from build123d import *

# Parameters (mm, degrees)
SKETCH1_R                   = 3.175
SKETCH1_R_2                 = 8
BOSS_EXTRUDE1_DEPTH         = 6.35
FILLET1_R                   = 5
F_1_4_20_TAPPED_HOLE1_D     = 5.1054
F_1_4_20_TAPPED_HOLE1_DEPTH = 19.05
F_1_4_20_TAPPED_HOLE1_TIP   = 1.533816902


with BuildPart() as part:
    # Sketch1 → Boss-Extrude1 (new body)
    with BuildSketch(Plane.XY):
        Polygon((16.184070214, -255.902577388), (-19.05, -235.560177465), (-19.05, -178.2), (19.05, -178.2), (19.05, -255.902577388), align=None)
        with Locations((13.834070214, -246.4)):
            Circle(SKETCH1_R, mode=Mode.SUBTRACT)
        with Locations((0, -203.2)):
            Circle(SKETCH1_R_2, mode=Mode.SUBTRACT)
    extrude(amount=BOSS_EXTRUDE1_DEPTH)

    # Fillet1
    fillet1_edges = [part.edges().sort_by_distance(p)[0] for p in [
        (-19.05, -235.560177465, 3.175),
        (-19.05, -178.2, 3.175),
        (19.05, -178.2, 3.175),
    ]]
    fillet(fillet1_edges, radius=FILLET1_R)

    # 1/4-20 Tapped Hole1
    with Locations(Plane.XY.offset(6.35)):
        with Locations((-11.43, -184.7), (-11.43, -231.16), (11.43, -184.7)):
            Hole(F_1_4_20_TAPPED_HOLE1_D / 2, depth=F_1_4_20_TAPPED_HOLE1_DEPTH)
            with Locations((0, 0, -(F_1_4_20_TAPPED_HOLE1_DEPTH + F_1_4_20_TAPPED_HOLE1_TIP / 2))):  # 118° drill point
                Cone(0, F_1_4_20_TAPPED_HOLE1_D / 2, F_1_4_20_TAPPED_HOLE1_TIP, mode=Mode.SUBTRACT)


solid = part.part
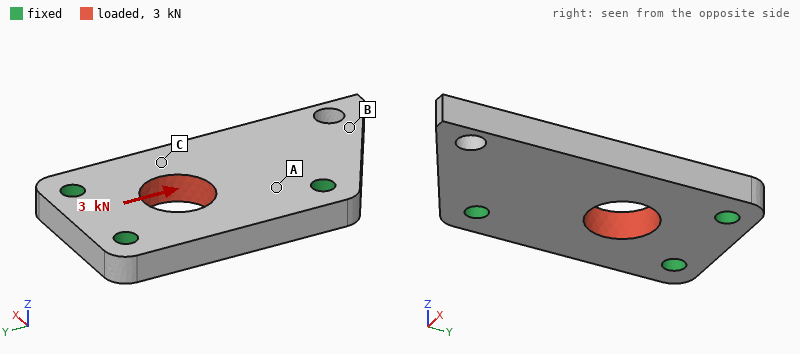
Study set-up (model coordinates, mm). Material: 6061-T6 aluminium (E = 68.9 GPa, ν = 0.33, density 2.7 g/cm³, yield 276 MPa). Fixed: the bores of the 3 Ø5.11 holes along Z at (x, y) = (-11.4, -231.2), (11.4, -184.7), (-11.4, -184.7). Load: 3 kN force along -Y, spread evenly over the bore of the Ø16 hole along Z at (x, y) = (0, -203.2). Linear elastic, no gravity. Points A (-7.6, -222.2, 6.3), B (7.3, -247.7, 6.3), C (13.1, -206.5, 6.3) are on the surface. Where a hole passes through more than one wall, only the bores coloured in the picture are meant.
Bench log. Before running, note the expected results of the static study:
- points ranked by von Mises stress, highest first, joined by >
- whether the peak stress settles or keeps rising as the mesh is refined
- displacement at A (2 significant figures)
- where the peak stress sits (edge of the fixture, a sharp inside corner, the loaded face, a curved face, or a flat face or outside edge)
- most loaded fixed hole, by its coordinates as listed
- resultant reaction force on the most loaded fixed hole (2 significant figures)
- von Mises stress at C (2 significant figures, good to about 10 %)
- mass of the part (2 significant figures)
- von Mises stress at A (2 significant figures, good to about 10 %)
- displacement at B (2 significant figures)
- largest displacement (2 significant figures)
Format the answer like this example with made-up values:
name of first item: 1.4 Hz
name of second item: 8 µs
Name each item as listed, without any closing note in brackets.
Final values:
points ranked by von Mises stress, highest first, joined by >: A > C > B
whether the peak stress settles or keeps rising as the mesh is refined: keeps rising
displacement at A: 1.5 µm
where the peak stress sits: edge of the fixture
most loaded fixed hole, by its coordinates as listed: (11.4, -184.7)
resultant reaction force on the most loaded fixed hole: 1.2 kN
von Mises stress at C: 5.2 MPa
mass of the part: 39 g
von Mises stress at A: 9.6 MPa
displacement at B: 3.5 µm
largest displacement: 5.1 µm
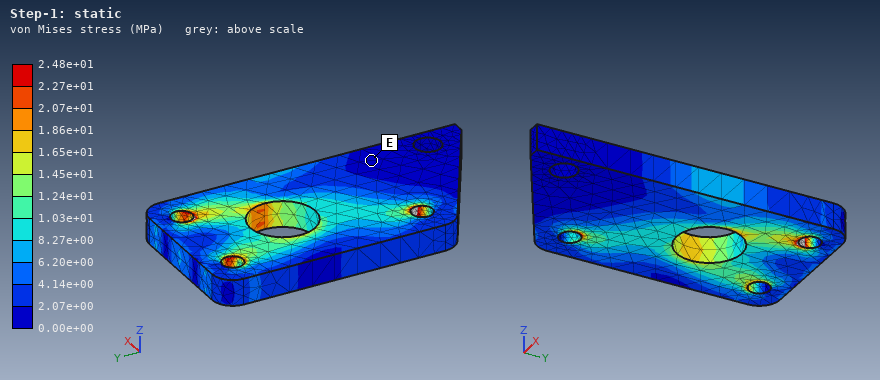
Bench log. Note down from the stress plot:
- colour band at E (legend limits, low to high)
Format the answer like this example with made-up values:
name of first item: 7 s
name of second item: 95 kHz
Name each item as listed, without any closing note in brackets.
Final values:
colour band at E: 0.00e+00 to 2.07e+00 MPa
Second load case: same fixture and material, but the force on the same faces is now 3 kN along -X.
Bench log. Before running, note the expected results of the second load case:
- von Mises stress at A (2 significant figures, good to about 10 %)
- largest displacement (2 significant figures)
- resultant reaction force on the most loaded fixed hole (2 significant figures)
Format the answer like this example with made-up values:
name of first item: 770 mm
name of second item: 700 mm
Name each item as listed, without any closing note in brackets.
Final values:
von Mises stress at A: 12 MPa
largest displacement: 8.7 µm
resultant reaction force on the most loaded fixed hole: 1.2 kN
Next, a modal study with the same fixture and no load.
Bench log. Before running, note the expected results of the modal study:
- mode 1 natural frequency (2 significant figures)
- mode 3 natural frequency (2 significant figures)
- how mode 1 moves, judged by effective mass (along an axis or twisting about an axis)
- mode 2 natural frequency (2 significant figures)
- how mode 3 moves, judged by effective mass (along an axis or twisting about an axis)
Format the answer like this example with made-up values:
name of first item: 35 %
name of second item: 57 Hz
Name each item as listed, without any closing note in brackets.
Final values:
mode 1 natural frequency: 4900 Hz
mode 3 natural frequency: 16 kHz
how mode 1 moves, judged by effective mass: along Z
mode 2 natural frequency: 9100 Hz
how mode 3 moves, judged by effective mass: along Z
